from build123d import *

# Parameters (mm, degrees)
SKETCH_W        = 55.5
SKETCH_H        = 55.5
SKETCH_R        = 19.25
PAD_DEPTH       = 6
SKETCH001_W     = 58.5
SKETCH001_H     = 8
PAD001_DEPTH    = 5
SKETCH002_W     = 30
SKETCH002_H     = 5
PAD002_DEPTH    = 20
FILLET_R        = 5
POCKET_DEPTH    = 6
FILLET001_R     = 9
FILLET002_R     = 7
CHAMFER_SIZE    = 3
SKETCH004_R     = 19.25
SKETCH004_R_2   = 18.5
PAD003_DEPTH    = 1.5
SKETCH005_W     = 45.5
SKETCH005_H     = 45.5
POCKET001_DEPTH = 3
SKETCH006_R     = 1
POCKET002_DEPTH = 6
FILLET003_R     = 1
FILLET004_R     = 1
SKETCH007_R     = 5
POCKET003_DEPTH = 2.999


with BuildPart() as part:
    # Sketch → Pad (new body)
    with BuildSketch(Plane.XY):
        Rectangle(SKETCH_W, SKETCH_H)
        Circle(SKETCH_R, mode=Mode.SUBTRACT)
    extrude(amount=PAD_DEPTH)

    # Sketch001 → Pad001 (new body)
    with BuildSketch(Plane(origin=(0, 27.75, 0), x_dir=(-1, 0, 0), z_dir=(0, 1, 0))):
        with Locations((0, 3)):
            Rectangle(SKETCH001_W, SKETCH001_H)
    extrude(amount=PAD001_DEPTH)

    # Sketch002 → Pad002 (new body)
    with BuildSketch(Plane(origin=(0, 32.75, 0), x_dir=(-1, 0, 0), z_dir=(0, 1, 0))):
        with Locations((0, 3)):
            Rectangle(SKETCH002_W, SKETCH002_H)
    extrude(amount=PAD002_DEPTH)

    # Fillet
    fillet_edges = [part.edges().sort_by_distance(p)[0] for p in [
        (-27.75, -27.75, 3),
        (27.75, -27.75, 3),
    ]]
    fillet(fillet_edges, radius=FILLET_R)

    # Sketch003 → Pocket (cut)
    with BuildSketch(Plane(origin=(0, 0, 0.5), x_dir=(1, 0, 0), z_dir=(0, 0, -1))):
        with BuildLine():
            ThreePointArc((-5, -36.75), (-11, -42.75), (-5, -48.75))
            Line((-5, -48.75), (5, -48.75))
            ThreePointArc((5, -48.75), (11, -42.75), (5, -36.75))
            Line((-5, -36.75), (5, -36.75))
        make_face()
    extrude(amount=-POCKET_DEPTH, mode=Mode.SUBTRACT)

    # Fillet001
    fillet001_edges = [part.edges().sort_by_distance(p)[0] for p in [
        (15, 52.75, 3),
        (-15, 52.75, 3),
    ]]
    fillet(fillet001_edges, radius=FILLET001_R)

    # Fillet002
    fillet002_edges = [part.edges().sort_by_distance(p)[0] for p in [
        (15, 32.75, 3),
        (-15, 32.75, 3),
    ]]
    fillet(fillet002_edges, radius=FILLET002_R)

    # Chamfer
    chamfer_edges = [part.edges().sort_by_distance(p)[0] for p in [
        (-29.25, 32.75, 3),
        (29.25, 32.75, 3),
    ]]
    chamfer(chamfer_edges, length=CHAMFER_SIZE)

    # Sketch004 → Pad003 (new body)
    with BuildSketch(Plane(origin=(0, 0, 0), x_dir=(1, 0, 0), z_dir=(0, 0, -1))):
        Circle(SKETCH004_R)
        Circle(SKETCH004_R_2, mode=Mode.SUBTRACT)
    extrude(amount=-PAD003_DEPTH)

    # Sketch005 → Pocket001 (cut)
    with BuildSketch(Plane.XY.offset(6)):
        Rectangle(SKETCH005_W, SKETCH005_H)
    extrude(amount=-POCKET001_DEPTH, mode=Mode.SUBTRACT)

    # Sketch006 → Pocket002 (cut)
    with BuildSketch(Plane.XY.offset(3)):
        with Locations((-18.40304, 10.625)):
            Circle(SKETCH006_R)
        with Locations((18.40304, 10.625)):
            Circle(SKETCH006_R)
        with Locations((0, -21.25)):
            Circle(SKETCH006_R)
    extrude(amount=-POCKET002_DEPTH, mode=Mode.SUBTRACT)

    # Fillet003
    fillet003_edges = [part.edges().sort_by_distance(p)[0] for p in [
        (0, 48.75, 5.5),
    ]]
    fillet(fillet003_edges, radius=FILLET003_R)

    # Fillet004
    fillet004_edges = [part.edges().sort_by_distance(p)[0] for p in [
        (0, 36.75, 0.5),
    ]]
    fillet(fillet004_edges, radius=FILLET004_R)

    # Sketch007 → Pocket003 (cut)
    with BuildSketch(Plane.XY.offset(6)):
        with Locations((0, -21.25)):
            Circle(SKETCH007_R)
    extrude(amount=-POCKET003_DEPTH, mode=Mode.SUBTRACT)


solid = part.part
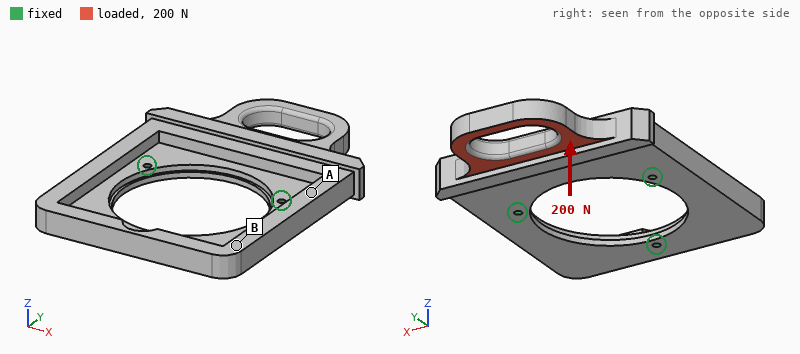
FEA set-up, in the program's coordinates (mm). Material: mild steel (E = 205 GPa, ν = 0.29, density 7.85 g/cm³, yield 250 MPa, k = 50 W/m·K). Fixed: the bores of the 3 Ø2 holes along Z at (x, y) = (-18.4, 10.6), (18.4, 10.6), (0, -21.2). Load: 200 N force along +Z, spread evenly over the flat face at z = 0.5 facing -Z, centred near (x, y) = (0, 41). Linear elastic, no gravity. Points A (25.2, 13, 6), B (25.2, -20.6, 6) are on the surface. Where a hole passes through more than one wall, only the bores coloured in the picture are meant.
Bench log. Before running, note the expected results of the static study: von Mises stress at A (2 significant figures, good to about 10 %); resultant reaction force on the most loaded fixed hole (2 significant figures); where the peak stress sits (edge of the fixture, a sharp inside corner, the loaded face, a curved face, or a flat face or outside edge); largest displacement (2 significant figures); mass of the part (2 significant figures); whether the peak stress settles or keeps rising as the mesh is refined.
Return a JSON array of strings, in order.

["58 MPa", "150 N", "edge of the fixture", "95 µm", "100 g", "keeps rising"]
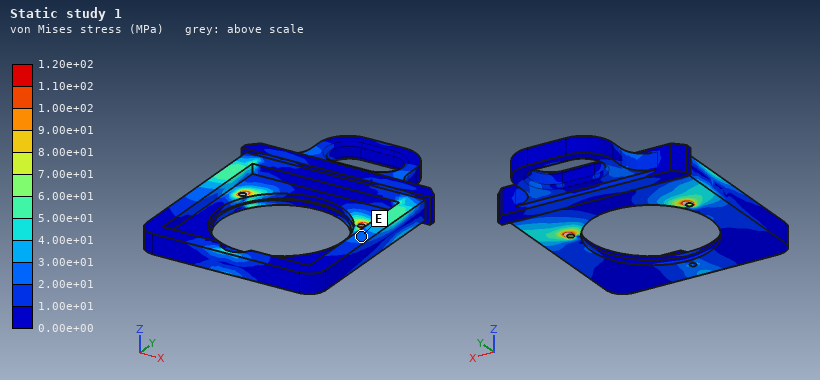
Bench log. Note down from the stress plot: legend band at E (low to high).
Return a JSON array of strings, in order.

["2.00e+01 to 3.00e+01 MPa"]
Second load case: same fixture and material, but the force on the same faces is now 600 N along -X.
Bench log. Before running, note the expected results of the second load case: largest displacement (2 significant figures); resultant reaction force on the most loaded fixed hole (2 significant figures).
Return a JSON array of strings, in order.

["11 µm", "520 N"]
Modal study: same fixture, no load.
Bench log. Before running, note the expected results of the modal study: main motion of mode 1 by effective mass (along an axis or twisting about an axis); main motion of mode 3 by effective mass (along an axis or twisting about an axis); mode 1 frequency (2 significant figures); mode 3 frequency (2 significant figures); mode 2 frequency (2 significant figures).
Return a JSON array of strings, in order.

["along Z", "along Z", "1800 Hz", "4900 Hz", "3400 Hz"]
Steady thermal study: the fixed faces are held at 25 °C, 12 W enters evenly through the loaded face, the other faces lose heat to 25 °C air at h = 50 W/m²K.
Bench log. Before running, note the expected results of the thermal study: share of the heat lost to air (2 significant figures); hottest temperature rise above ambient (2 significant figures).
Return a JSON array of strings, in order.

["45 %", "59 K"]
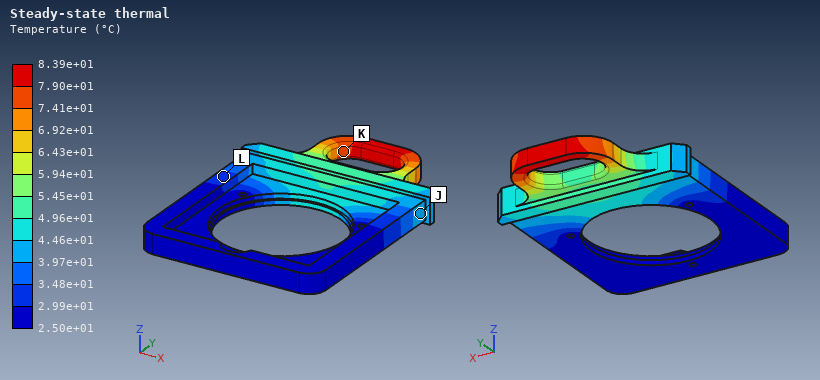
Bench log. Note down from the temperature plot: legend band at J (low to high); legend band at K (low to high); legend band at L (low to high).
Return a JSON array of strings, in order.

["3.97e+01 to 4.46e+01 °C", "7.41e+01 to 7.90e+01 °C", "2.99e+01 to 3.48e+01 °C"]
